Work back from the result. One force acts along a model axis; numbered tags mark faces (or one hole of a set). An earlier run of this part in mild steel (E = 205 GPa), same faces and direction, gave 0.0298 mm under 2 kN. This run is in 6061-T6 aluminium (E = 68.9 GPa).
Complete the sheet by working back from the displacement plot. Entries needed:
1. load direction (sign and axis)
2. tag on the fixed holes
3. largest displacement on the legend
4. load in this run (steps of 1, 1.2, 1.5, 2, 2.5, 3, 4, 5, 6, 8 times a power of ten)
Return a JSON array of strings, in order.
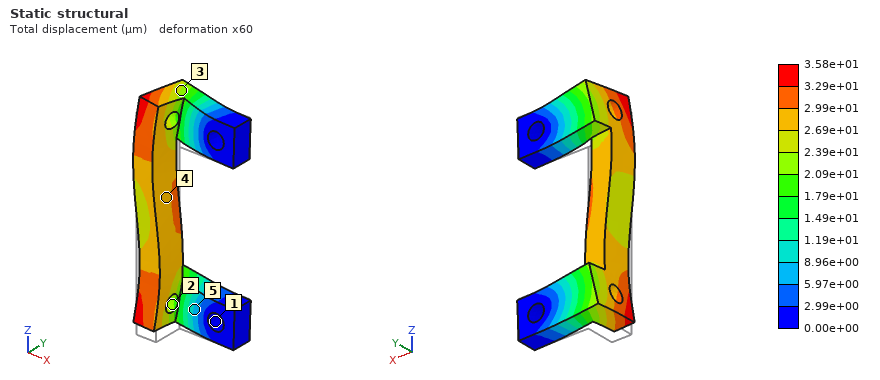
["+Z", "1", "3.58e+01 µm", "800 N"]
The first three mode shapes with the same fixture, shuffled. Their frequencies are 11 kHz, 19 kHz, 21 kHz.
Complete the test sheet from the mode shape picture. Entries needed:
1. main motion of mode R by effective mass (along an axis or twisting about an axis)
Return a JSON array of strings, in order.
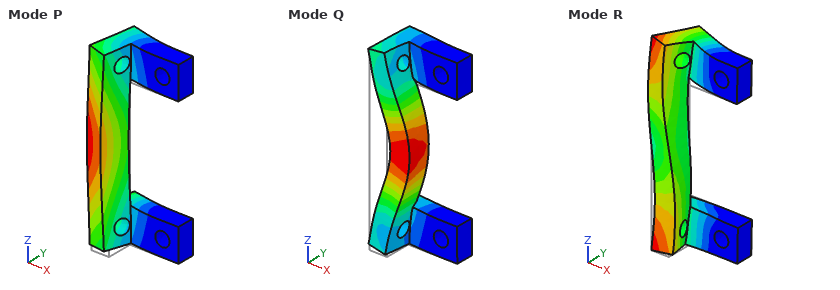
["along Z"]
